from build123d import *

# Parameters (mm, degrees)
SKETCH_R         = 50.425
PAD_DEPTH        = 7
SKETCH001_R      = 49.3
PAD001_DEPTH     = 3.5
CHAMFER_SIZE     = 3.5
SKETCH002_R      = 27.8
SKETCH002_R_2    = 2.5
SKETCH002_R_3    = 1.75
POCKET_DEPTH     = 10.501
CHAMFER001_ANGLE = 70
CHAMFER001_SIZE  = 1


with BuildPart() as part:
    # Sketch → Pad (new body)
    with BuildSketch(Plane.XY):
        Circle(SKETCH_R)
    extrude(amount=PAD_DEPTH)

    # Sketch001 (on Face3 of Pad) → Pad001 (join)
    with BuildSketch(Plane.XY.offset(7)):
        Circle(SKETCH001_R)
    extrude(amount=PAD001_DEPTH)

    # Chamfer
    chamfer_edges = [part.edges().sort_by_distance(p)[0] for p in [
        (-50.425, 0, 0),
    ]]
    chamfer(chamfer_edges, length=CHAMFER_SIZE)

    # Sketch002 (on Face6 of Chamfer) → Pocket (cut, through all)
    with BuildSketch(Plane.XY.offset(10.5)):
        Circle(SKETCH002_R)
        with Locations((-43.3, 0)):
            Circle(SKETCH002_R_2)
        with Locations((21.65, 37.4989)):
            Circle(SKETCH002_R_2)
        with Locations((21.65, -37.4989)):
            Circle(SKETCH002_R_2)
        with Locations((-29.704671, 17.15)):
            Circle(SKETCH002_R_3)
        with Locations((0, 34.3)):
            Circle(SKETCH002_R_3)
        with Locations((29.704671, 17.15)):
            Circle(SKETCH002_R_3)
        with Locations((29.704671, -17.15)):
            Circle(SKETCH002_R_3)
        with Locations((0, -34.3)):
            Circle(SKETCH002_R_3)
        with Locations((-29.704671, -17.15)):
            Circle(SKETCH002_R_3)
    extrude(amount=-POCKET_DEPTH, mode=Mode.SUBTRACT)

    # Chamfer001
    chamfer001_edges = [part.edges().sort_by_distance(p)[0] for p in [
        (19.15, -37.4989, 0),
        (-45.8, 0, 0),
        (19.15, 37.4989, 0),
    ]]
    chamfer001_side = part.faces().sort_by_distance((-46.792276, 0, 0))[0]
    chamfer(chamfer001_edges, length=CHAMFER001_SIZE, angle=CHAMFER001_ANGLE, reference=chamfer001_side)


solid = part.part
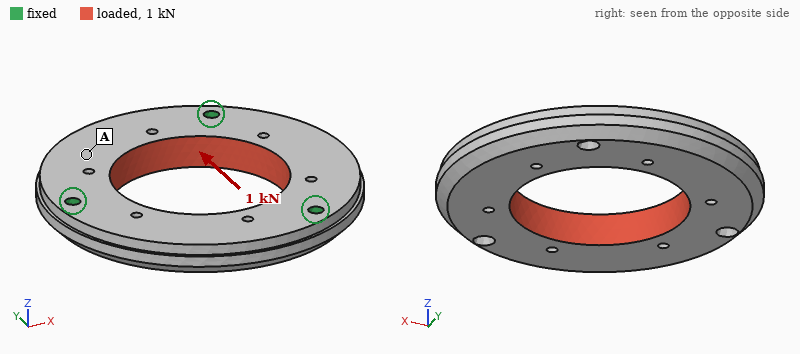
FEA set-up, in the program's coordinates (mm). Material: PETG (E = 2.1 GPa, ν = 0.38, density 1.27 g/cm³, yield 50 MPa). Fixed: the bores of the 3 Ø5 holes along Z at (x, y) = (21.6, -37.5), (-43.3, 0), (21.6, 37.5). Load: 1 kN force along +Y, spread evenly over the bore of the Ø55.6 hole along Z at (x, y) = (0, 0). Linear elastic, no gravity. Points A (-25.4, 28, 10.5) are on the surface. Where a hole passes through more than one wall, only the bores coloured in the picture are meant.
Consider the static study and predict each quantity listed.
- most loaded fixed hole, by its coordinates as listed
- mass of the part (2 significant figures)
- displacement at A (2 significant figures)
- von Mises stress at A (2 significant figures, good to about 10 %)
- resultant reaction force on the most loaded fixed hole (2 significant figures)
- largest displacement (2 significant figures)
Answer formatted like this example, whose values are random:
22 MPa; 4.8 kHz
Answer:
(-43.3, 0); 69 g; 33 µm; 0.86 MPa; 430 N; 41 µm
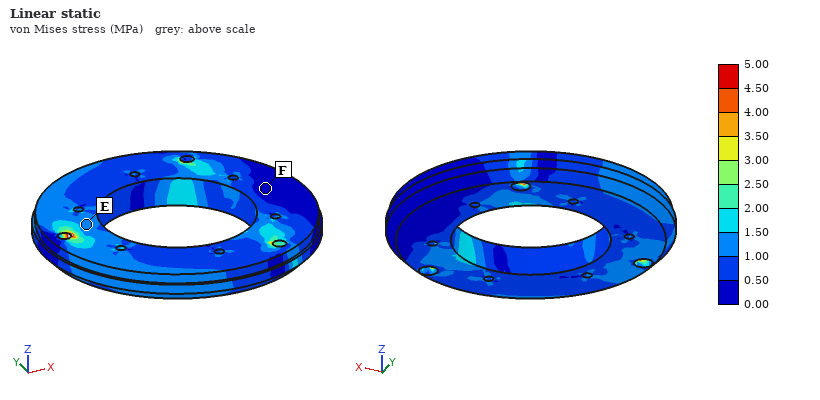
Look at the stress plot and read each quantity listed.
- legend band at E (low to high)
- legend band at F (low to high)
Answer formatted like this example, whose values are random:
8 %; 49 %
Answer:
1.00 to 1.50 MPa; 0.00 to 0.50 MPa
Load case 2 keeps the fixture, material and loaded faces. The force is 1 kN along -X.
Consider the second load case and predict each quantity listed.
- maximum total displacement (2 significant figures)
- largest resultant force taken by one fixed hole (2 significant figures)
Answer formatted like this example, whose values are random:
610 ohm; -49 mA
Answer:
47 µm; 390 N
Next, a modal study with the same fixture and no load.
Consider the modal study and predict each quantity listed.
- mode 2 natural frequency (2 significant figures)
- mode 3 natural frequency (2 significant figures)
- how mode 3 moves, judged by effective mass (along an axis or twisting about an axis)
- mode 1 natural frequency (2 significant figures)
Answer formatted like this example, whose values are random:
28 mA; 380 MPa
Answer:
1300 Hz; 1600 Hz; along Z; 1300 Hz
